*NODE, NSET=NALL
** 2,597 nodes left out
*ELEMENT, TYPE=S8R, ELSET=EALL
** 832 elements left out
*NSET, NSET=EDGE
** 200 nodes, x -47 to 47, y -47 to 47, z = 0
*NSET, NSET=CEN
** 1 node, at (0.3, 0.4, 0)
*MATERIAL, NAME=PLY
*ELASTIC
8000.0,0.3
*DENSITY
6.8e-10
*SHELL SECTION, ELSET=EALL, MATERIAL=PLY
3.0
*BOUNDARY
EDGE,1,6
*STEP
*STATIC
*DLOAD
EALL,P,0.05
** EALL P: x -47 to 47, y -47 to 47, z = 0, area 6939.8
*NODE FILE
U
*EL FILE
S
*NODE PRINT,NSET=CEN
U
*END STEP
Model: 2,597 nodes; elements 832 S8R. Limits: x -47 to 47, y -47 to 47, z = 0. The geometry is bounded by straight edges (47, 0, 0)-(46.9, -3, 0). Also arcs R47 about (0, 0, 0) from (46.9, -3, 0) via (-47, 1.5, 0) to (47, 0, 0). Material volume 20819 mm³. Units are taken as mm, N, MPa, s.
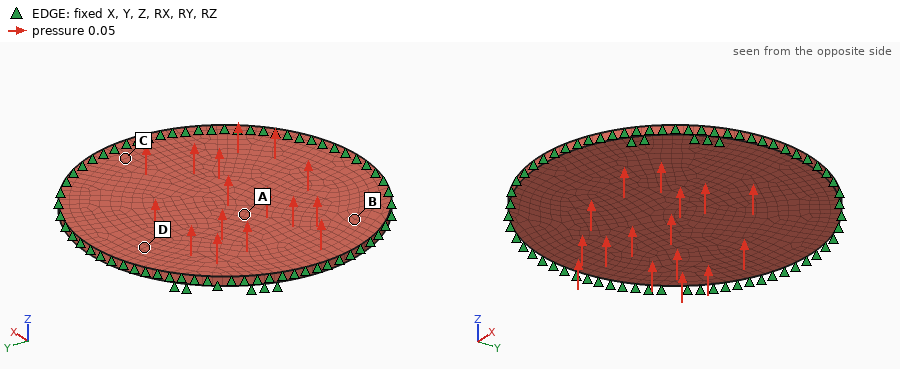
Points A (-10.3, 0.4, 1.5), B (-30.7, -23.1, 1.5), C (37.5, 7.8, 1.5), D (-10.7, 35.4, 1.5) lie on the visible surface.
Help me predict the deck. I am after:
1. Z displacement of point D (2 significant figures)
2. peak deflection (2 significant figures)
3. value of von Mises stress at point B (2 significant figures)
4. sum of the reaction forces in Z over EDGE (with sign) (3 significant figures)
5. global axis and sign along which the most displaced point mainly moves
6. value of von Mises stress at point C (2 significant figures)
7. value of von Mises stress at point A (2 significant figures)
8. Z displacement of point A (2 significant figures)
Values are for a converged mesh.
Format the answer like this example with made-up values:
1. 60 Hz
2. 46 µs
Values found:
1. 0.029 mm
2. 0.19 mm
3. 4.3 MPa
4. -347 N
5. +Z
6. 4.2 MPa
7. 5.4 MPa
8. 0.18 mm
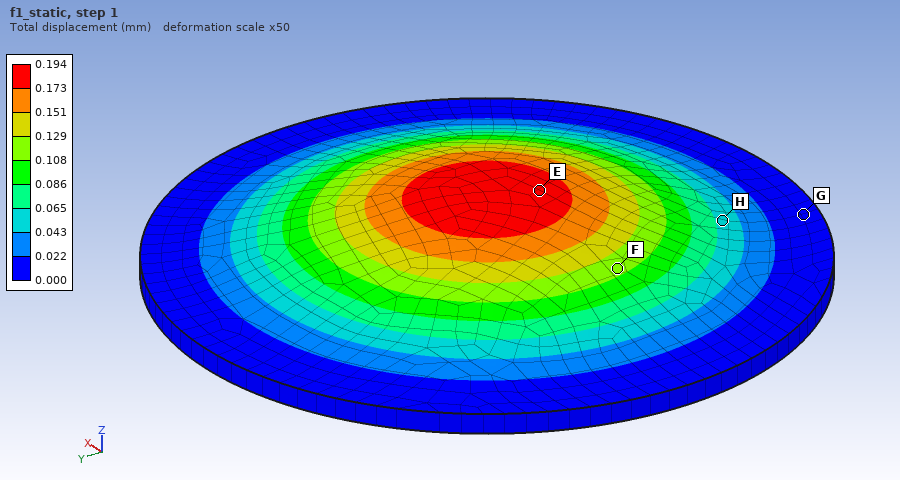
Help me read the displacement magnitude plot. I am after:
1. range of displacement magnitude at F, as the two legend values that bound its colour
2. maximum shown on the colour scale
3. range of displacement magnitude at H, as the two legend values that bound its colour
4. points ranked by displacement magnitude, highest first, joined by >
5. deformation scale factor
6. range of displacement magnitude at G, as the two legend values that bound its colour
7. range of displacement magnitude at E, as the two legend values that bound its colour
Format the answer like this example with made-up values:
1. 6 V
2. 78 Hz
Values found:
1. 0.108 to 0.129 mm
2. 0.194 mm
3. 0.043 to 0.065 mm
4. E > F > H > G
5. 50
6. 0.000 to 0.022 mm
7. 0.173 to 0.194 mm
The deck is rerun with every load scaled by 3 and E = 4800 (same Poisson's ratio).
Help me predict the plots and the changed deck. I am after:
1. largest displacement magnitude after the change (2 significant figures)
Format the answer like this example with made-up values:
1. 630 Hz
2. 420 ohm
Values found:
1. 0.97 mm
